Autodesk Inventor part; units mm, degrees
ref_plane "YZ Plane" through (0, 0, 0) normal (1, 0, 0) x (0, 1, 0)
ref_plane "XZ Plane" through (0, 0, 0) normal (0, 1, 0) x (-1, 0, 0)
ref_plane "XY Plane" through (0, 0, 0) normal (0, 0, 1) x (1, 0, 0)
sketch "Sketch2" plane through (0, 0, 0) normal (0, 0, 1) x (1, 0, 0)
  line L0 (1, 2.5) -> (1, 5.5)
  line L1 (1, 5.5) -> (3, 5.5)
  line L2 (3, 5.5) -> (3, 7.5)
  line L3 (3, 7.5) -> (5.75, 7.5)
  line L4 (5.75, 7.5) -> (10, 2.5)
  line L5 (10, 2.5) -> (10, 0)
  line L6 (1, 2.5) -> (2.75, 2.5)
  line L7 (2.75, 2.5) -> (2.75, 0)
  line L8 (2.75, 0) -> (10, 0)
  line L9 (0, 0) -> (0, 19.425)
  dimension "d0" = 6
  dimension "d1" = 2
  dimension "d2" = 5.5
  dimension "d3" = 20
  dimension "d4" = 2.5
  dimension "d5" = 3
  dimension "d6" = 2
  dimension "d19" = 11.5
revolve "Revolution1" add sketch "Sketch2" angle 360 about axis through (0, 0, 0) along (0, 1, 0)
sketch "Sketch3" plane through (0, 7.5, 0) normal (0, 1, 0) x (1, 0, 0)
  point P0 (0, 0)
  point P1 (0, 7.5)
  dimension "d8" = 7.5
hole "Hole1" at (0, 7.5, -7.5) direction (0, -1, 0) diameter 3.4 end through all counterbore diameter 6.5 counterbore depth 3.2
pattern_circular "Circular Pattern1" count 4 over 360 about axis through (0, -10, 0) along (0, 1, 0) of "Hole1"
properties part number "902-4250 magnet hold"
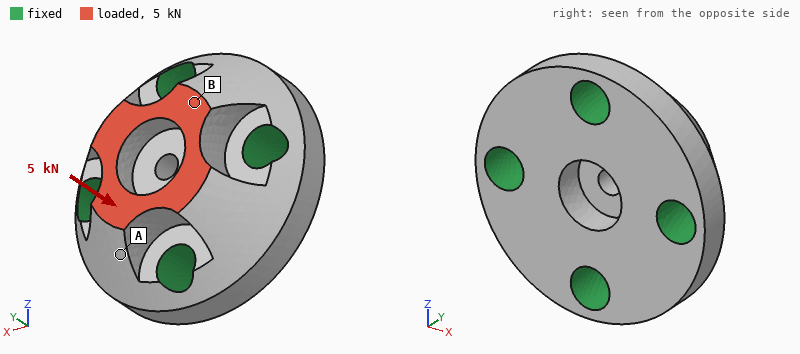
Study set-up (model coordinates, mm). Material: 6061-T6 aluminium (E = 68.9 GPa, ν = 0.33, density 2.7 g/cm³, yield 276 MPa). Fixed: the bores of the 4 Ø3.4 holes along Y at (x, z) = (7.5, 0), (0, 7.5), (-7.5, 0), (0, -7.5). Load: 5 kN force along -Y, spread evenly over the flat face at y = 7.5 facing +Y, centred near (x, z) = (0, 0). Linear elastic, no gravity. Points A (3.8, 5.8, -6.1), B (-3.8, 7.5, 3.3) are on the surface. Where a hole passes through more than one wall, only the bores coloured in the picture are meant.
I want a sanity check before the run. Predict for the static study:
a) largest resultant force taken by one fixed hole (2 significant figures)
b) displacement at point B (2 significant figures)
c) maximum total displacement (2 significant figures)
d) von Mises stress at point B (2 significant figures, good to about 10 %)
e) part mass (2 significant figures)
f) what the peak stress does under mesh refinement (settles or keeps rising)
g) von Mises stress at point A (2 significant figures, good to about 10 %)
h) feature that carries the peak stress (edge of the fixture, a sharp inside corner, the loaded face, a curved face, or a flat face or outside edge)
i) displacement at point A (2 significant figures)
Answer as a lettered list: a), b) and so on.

a) 1.3 kN
b) 7.2 µm
c) 8.9 µm
d) 54 MPa
e) 3.6 g
f) keeps rising
g) 25 MPa
h) edge of the fixture
i) 2.9 µm
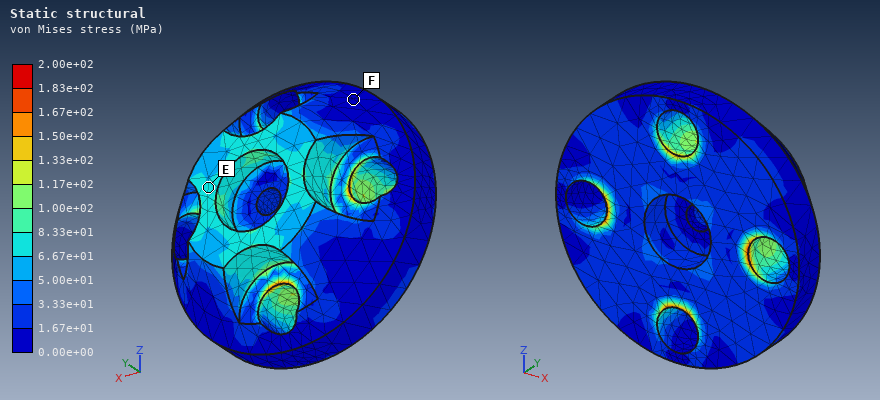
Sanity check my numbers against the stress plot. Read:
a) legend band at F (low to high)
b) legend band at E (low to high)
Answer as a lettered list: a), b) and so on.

a) 0.00e+00 to 1.67e+01 MPa
b) 6.67e+01 to 8.33e+01 MPa
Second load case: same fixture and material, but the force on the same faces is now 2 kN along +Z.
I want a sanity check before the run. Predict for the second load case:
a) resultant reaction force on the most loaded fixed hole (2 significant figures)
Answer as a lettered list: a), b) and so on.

a) 870 N
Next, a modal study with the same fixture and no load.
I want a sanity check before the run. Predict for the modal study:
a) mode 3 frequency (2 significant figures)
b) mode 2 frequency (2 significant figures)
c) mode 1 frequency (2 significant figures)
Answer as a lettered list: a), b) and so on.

a) 110 kHz
b) 110 kHz
c) 110 kHz
